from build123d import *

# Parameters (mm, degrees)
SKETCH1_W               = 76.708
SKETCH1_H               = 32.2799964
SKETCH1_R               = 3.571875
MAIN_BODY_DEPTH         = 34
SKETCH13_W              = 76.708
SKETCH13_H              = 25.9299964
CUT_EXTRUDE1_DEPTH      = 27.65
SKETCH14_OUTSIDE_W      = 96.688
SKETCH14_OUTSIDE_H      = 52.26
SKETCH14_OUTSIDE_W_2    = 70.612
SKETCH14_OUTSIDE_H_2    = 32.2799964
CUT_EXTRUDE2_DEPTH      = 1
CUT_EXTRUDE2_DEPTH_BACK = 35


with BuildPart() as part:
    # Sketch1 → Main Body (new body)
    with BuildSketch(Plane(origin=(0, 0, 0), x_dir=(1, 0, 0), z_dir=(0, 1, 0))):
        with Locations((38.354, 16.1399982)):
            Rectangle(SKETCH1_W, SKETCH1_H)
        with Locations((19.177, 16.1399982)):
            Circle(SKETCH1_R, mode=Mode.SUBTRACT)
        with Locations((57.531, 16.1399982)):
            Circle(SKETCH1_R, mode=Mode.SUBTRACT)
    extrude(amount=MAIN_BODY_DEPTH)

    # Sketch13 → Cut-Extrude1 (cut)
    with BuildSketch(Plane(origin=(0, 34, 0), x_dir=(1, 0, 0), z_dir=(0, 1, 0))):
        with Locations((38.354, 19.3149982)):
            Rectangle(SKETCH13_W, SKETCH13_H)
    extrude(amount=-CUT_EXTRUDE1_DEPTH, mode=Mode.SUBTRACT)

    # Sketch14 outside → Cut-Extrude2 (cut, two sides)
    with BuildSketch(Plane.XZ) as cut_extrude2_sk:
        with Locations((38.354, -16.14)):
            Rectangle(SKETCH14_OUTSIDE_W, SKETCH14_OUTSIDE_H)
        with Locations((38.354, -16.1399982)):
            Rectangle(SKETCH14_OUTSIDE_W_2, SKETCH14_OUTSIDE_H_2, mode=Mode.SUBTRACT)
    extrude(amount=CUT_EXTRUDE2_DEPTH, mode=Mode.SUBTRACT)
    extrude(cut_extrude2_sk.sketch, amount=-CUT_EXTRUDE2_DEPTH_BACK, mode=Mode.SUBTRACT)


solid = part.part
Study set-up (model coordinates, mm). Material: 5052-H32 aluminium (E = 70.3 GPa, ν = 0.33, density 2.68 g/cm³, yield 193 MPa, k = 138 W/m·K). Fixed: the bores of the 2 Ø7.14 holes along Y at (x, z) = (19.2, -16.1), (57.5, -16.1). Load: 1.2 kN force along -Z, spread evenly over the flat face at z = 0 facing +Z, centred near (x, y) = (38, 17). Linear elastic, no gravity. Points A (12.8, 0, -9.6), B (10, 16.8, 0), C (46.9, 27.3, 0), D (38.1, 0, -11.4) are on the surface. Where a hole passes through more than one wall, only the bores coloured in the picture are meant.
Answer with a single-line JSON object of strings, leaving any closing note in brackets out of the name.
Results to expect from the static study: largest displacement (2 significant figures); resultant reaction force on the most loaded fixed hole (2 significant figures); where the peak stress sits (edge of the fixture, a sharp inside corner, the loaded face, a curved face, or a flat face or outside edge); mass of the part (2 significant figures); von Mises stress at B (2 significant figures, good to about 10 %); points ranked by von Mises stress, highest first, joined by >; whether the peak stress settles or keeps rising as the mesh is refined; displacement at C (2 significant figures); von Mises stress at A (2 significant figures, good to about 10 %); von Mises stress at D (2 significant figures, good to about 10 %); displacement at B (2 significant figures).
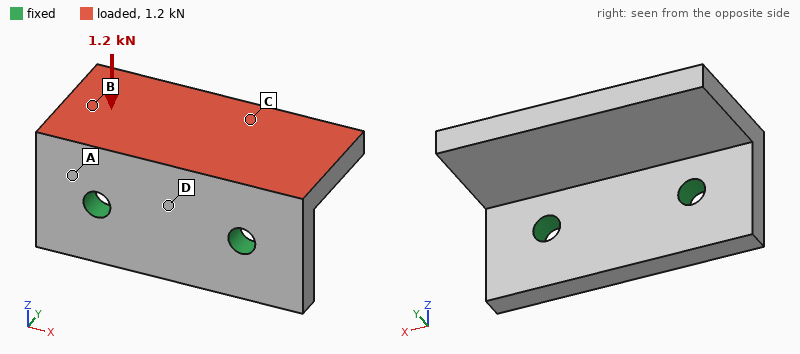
{"largest displacement": "89 µm", "resultant reaction force on the most loaded fixed hole": "600 N", "where the peak stress sits": "edge of the fixture", "mass of the part": "71 g", "von Mises stress at B": "11 MPa", "points ranked by von Mises stress, highest first, joined by >": "A > D > B > C", "whether the peak stress settles or keeps rising as the mesh is refined": "keeps rising", "displacement at C": "69 µm", "von Mises stress at A": "27 MPa", "von Mises stress at D": "19 MPa", "displacement at B": "39 µm"}
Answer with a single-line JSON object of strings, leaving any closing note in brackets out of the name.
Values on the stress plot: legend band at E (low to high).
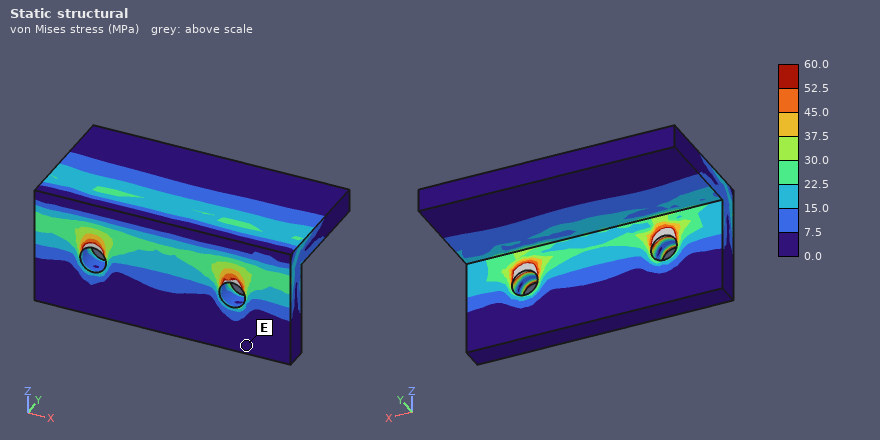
{"legend band at E": "0.0 to 7.5 MPa"}
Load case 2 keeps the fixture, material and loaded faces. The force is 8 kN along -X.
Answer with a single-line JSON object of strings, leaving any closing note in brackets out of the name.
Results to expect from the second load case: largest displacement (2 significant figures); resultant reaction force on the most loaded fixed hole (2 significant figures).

{"largest displacement": "76 µm", "resultant reaction force on the most loaded fixed hole": "5.4 kN"}
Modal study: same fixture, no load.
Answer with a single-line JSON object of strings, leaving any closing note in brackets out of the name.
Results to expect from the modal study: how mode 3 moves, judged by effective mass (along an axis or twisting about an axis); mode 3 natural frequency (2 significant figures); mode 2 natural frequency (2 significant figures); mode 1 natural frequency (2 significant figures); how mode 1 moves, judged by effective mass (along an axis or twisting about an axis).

{"how mode 3 moves, judged by effective mass": "along X", "mode 3 natural frequency": "9200 Hz", "mode 2 natural frequency": "5500 Hz", "mode 1 natural frequency": "3500 Hz", "how mode 1 moves, judged by effective mass": "along Z"}
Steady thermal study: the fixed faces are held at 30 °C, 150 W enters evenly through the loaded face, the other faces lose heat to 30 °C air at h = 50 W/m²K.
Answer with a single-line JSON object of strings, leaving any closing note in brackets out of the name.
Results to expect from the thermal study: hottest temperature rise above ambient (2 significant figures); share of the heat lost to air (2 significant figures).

{"hottest temperature rise above ambient": "61 K", "share of the heat lost to air": "6.9 %"}
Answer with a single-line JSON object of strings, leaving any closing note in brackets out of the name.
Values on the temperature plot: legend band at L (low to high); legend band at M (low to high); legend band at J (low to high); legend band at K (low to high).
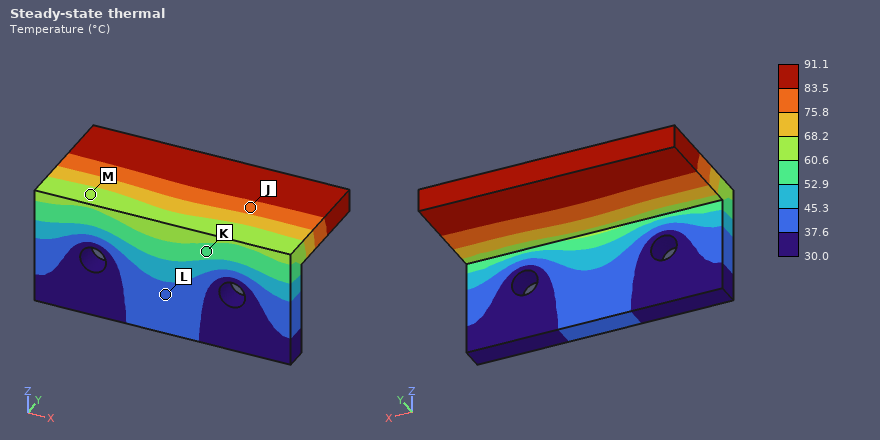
{"legend band at L": "37.6 to 45.3 °C", "legend band at M": "60.6 to 68.2 °C", "legend band at J": "75.8 to 83.5 °C", "legend band at K": "52.9 to 60.6 °C"}
